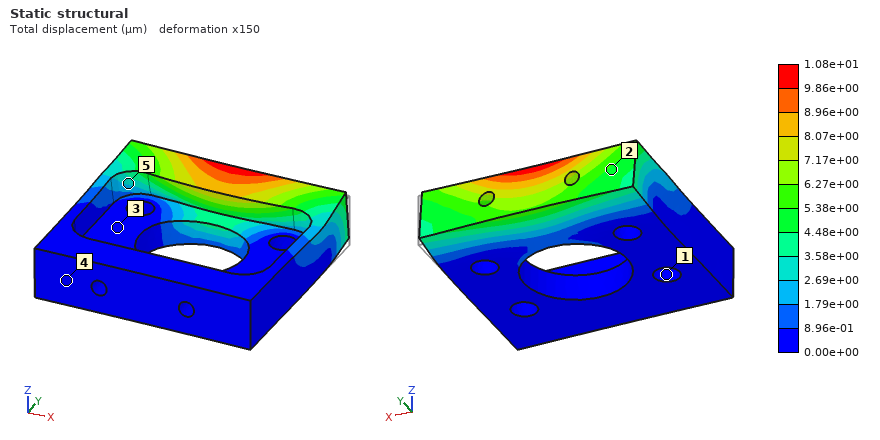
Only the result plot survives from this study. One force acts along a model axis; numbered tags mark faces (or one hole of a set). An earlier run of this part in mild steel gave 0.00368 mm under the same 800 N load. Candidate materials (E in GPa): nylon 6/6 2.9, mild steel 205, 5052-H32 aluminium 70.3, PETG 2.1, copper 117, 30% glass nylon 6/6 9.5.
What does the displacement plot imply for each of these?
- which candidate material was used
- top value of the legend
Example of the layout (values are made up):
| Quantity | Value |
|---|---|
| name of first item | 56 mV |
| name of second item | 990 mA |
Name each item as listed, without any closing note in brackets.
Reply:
| Quantity | Value |
|---|---|
| which candidate material was used | 5052-H32 aluminium |
| top value of the legend | 1.08e+01 µm |
